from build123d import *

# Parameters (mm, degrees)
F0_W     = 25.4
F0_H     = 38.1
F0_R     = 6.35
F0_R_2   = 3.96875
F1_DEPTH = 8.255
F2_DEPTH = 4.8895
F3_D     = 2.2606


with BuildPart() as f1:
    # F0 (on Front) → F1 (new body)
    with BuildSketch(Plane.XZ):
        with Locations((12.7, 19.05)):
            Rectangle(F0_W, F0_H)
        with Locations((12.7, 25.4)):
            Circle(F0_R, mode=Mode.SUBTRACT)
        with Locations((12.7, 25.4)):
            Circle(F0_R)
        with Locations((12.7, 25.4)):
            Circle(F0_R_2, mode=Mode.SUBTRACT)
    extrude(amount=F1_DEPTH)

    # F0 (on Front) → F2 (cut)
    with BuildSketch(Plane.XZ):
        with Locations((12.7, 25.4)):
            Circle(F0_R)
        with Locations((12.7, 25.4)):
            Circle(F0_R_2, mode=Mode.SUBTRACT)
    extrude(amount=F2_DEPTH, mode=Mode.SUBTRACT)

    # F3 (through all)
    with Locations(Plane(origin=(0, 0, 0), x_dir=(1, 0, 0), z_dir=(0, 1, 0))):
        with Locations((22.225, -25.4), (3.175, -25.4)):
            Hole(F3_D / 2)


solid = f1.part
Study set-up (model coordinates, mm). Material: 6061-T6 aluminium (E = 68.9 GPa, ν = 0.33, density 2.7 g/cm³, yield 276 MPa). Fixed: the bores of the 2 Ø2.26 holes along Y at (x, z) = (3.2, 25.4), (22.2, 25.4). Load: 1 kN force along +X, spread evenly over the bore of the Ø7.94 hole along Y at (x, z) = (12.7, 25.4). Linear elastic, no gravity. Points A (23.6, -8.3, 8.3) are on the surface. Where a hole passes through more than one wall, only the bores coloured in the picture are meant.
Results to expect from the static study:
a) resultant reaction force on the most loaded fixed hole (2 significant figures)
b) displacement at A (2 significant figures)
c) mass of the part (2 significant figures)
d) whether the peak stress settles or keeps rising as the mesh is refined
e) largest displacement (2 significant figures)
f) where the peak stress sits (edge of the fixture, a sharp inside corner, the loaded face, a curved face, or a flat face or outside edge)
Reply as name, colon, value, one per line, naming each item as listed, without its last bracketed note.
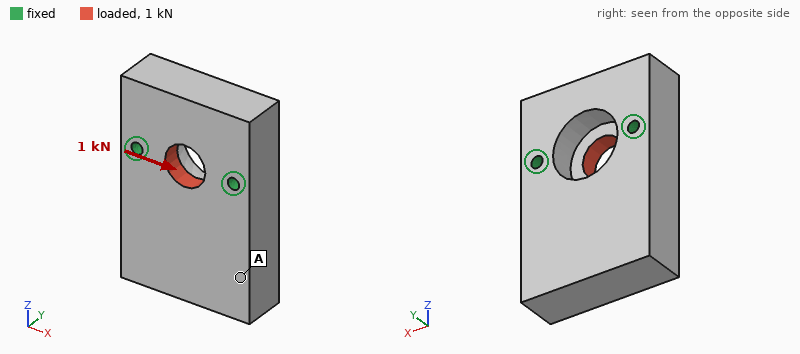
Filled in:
resultant reaction force on the most loaded fixed hole: 500 N
displacement at A: 1.0 µm
mass of the part: 19 g
whether the peak stress settles or keeps rising as the mesh is refined: keeps rising
largest displacement: 1.8 µm
where the peak stress sits: edge of the fixture
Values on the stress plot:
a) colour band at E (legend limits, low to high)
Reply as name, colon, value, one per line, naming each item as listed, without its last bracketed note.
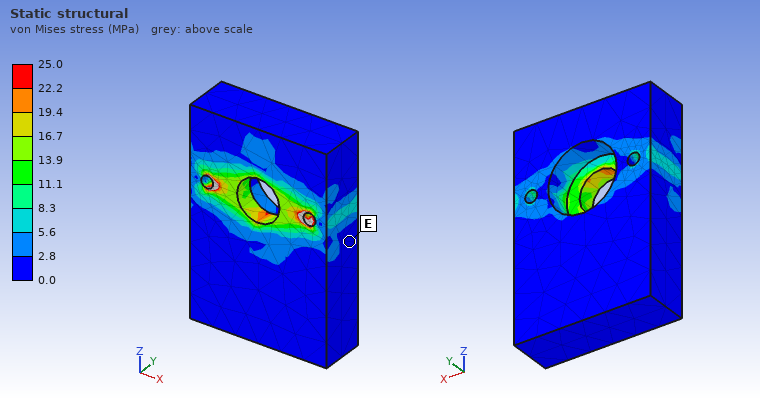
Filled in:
colour band at E: 0.0 to 2.8 MPa
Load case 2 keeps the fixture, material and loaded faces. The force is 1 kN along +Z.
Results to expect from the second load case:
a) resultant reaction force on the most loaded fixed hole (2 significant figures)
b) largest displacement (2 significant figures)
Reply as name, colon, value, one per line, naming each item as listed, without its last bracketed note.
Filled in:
resultant reaction force on the most loaded fixed hole: 500 N
largest displacement: 4.6 µm
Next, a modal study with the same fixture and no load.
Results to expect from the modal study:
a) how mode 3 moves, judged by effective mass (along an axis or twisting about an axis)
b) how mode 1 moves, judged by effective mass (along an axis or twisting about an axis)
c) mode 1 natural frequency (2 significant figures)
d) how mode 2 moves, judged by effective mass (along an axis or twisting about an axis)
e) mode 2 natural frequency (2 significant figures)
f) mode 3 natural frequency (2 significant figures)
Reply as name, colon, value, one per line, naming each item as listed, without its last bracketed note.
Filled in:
how mode 3 moves, judged by effective mass: along X
how mode 1 moves, judged by effective mass: along Y
mode 1 natural frequency: 7800 Hz
how mode 2 moves, judged by effective mass: along X
mode 2 natural frequency: 18 kHz
mode 3 natural frequency: 19 kHz
